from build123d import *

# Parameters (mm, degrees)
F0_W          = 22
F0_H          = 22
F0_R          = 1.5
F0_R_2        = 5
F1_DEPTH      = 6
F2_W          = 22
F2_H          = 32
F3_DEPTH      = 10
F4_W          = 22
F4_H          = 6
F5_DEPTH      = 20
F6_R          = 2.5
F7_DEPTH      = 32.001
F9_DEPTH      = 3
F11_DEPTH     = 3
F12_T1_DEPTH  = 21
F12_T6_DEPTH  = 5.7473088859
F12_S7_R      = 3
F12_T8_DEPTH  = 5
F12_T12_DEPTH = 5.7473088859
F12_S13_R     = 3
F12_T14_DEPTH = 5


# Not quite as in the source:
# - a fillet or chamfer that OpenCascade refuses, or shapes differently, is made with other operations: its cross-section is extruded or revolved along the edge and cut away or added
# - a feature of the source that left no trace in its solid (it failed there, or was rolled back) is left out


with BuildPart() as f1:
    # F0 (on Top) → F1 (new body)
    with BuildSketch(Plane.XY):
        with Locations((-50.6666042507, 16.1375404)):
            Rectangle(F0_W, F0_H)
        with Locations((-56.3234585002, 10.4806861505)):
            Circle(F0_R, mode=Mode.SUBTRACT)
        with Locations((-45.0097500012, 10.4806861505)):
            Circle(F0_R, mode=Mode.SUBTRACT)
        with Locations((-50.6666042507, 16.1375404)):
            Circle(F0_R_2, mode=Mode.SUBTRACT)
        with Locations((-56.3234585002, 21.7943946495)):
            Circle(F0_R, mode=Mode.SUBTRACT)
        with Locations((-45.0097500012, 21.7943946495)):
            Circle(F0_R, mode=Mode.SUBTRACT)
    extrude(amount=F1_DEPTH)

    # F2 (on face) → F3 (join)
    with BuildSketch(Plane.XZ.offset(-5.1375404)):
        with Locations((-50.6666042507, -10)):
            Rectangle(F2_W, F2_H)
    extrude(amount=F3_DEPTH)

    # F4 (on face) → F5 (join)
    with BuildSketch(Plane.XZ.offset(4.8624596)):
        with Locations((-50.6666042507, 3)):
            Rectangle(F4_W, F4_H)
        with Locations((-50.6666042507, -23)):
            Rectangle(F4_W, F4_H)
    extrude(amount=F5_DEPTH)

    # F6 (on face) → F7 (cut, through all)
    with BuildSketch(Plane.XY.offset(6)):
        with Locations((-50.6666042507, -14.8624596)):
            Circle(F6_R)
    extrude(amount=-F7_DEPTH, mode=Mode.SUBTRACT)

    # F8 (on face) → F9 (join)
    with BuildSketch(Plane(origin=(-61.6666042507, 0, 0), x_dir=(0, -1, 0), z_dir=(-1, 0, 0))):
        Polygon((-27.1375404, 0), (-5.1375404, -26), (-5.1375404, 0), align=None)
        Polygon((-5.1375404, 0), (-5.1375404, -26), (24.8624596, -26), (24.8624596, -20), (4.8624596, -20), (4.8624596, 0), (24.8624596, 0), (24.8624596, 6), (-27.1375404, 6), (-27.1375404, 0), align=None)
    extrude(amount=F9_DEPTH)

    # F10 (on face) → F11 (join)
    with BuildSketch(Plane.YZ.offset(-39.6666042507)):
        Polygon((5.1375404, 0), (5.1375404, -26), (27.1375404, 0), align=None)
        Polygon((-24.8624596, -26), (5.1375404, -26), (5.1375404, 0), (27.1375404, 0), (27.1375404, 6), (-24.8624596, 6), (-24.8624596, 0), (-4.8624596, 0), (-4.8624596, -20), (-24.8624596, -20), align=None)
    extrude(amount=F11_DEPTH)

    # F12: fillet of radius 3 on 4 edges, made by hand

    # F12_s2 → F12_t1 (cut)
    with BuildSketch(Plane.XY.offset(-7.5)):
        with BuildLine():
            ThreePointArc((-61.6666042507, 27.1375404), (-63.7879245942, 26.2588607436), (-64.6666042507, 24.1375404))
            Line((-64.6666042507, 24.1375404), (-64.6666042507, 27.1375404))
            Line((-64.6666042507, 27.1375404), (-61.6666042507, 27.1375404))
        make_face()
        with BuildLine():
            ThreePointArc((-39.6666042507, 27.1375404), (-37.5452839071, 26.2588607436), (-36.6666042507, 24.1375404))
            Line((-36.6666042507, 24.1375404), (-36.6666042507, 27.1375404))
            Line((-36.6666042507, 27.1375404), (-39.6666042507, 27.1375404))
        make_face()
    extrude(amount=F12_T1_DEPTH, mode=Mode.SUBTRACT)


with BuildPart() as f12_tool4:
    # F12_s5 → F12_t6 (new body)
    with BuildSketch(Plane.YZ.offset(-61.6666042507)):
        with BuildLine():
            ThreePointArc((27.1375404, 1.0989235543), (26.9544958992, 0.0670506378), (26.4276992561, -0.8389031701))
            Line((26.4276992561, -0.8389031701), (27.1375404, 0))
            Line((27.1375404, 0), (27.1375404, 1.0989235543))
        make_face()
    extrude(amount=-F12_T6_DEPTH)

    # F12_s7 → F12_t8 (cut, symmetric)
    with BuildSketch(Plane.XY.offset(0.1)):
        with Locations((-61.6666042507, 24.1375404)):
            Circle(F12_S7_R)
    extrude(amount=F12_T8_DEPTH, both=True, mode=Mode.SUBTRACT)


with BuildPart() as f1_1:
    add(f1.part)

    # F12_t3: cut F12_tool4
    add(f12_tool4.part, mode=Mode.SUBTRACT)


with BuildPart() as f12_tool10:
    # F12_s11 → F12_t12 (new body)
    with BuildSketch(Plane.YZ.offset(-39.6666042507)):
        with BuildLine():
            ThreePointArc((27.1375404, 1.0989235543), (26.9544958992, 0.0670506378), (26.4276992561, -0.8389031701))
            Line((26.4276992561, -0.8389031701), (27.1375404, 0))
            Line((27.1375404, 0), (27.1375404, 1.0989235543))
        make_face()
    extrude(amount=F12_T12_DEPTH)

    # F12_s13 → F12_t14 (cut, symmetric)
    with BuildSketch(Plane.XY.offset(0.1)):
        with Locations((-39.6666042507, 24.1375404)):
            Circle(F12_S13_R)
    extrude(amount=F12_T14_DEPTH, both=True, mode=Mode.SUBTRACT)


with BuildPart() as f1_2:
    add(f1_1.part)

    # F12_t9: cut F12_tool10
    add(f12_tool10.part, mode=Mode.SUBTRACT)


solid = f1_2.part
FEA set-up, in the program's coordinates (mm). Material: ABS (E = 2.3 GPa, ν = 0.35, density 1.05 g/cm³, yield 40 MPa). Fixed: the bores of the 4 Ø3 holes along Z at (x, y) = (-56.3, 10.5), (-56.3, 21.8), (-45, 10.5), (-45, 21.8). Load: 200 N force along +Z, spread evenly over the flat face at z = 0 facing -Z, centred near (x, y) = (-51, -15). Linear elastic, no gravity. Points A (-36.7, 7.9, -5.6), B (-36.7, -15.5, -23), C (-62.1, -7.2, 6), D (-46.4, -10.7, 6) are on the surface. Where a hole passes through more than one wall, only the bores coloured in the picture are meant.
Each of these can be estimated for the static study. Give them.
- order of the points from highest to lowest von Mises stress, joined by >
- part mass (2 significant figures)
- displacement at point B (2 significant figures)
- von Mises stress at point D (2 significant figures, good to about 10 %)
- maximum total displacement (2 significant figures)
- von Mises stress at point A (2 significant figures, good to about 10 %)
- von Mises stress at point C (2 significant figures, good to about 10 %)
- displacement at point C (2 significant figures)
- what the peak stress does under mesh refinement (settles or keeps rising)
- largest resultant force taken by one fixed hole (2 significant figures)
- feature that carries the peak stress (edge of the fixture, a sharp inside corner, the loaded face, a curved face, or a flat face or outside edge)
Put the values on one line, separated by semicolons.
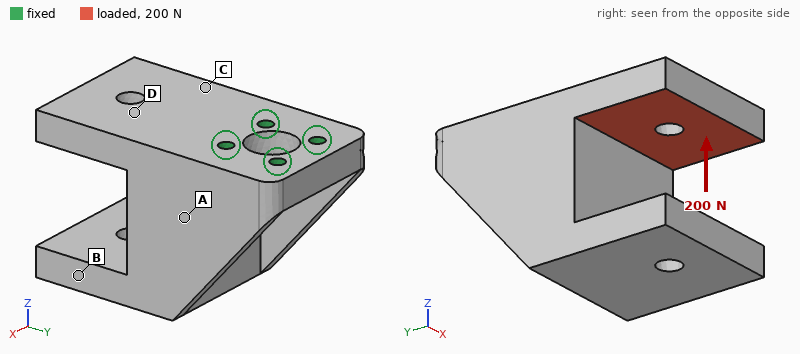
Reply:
C > D > A > B; 21 g; 0.31 mm; 6.0 MPa; 0.67 mm; 4.1 MPa; 8.9 MPa; 0.22 mm; keeps rising; 210 N; edge of the fixture
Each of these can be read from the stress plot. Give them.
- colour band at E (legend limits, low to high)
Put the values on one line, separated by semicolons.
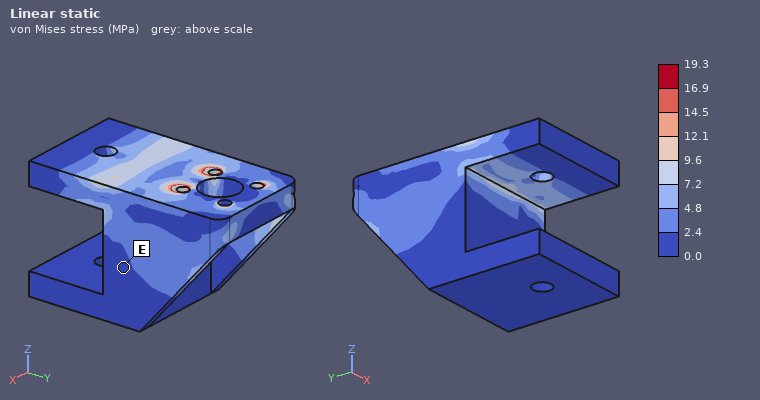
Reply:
0.0 to 2.4 MPa
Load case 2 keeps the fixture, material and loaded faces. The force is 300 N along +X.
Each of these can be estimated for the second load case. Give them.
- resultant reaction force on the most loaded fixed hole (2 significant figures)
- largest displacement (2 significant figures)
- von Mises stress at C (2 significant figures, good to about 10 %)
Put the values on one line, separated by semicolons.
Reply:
390 N; 0.25 mm; 3.8 MPa
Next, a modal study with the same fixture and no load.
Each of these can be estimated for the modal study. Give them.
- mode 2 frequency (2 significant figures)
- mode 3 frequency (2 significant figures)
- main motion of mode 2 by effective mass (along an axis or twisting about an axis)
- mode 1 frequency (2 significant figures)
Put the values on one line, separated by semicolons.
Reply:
1700 Hz; 2400 Hz; along X; 1100 Hz
